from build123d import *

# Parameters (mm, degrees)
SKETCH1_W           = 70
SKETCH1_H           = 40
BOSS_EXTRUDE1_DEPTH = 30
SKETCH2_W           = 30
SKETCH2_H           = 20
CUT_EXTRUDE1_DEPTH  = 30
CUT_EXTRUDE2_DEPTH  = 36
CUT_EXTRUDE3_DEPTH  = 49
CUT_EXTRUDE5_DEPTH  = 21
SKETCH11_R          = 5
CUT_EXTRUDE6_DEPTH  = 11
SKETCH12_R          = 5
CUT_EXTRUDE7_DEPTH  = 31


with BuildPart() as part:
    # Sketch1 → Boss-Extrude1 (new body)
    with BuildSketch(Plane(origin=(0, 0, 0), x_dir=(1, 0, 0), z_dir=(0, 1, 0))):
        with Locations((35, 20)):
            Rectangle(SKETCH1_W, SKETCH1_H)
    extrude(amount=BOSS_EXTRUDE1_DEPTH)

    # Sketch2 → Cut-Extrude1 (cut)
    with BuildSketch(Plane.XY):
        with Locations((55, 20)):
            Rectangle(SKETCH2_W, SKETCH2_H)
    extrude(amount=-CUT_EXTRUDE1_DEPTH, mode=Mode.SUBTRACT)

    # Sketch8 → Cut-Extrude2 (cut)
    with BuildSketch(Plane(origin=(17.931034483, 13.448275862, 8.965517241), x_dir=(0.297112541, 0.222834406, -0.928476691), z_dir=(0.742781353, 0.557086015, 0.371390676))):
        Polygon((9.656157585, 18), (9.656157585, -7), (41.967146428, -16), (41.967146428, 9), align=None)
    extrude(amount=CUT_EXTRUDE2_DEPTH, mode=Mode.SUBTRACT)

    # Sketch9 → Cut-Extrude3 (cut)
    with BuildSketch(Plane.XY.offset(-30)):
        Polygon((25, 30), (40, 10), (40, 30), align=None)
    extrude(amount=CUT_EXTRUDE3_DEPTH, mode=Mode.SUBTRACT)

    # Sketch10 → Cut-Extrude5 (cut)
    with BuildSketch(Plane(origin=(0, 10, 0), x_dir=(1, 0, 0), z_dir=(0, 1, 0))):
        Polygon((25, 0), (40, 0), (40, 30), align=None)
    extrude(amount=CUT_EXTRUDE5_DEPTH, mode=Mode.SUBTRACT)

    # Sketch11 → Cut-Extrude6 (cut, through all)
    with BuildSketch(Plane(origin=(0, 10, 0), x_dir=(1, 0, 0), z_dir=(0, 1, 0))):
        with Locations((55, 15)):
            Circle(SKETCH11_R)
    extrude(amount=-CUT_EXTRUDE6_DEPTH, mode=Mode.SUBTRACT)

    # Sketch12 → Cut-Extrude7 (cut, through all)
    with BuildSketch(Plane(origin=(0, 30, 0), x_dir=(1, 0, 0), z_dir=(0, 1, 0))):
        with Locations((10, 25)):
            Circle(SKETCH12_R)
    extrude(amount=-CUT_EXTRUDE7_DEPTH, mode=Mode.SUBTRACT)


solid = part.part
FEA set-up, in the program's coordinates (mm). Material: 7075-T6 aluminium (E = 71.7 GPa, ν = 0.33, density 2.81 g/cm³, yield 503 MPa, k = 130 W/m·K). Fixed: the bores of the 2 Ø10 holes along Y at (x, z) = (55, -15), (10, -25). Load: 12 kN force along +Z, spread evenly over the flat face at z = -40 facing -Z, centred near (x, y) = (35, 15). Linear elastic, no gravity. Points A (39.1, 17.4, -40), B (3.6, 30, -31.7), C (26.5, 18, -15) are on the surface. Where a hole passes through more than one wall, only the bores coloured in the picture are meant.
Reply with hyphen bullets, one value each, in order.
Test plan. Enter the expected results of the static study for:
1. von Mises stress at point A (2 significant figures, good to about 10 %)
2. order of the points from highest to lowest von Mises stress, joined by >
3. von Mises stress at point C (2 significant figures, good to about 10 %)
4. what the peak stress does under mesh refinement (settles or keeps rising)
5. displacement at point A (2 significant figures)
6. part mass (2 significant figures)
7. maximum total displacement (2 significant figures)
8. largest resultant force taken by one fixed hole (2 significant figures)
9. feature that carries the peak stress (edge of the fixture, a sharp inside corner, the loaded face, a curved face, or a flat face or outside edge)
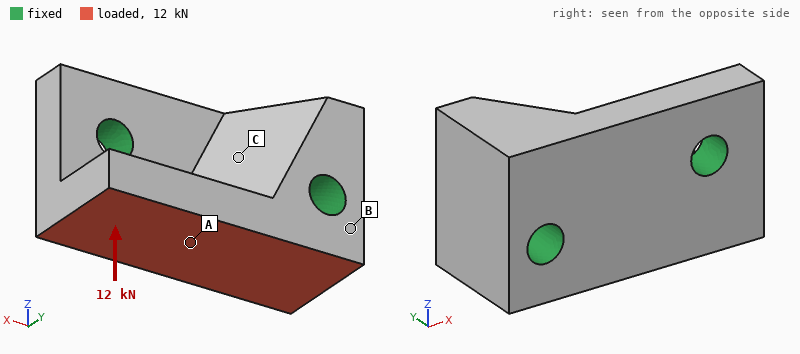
- 43 MPa
- A > C > B
- 12 MPa
- keeps rising
- 21 µm
- 150 g
- 80 µm
- 6.2 kN
- edge of the fixture
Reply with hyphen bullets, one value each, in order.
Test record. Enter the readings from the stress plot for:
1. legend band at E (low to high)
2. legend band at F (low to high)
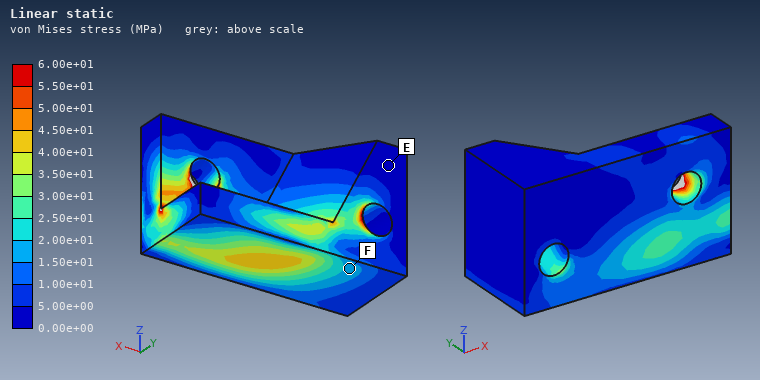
- 0.00e+00 to 5.00e+00 MPa
- 1.50e+01 to 2.00e+01 MPa
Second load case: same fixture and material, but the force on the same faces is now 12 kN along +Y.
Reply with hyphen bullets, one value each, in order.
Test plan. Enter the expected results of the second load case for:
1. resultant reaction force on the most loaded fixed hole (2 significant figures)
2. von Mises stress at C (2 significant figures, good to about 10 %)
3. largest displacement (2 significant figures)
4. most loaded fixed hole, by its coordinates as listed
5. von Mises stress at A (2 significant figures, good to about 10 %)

- 8.7 kN
- 13 MPa
- 0.11 mm
- (10, -25)
- 53 MPa
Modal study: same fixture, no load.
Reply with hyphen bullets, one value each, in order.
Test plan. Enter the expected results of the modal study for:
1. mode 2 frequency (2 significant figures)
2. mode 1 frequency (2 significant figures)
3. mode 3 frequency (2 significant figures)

- 16 kHz
- 9700 Hz
- 22 kHz
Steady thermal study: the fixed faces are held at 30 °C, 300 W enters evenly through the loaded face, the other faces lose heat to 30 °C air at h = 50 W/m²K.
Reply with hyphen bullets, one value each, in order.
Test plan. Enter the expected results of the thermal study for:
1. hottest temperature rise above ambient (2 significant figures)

- 66 K
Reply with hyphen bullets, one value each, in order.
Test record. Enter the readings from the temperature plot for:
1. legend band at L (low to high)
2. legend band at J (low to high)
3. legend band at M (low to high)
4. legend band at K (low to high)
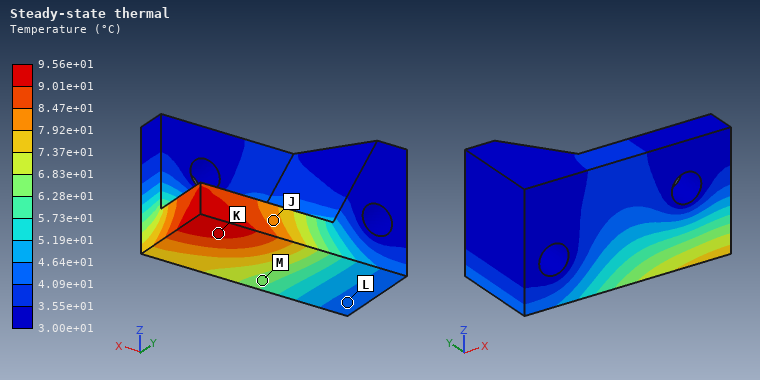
- 4.09e+01 to 4.64e+01 °C
- 7.92e+01 to 8.47e+01 °C
- 6.28e+01 to 6.83e+01 °C
- 9.01e+01 to 9.56e+01 °C
